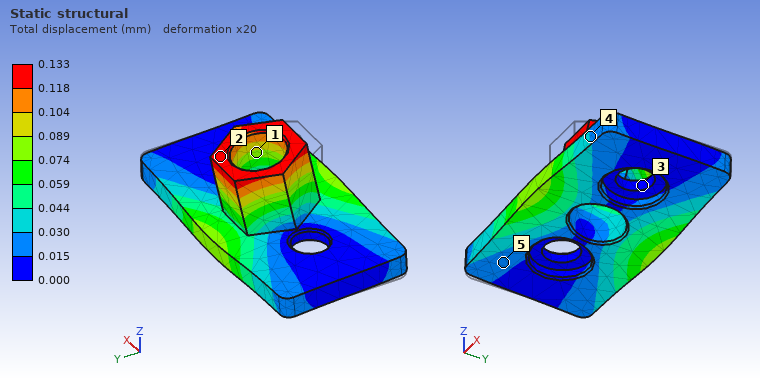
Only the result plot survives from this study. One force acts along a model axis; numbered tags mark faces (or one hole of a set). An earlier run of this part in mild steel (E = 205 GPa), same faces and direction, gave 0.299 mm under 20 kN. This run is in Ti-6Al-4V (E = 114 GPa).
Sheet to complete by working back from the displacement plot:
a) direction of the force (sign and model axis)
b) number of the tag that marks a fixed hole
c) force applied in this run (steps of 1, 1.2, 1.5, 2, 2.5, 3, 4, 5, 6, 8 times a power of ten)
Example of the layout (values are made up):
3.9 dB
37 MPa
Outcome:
+Y
3
5 kN
